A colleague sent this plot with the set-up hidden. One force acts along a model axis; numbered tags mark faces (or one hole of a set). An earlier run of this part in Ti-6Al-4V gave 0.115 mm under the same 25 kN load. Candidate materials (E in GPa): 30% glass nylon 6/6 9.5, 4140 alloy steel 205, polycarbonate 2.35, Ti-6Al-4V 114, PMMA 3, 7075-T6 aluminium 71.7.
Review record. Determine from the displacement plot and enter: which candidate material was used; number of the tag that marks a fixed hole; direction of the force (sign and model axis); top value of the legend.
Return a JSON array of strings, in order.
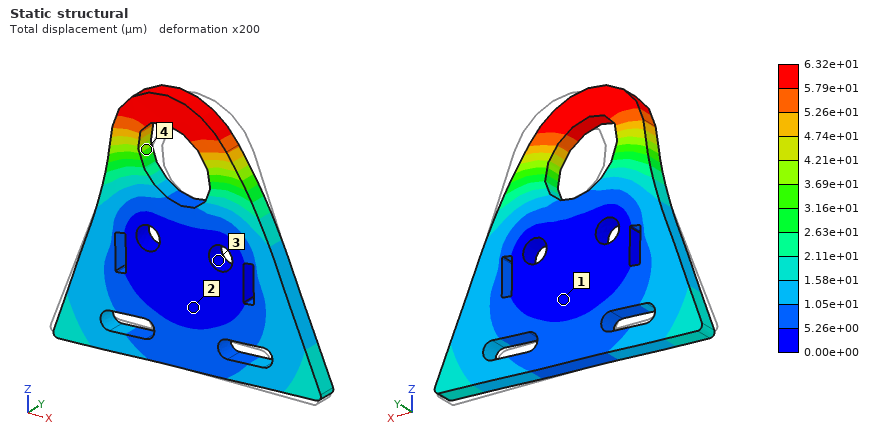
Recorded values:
["4140 alloy steel", "3", "-X", "6.32e+01 µm"]
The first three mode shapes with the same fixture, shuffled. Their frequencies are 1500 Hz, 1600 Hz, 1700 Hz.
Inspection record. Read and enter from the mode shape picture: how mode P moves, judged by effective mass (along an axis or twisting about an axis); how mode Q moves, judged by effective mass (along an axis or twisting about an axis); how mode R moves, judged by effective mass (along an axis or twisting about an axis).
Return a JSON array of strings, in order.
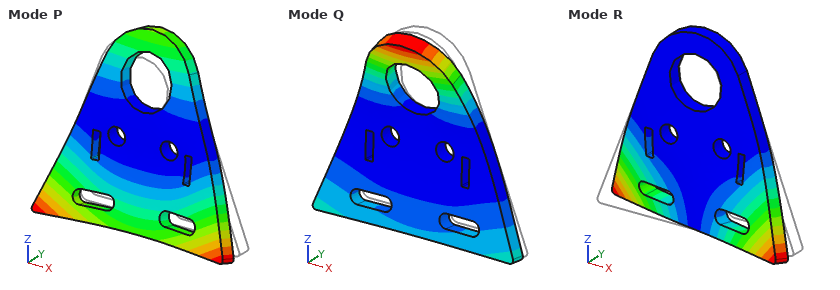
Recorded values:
["along Y", "along Y", "twisting about Z"]
